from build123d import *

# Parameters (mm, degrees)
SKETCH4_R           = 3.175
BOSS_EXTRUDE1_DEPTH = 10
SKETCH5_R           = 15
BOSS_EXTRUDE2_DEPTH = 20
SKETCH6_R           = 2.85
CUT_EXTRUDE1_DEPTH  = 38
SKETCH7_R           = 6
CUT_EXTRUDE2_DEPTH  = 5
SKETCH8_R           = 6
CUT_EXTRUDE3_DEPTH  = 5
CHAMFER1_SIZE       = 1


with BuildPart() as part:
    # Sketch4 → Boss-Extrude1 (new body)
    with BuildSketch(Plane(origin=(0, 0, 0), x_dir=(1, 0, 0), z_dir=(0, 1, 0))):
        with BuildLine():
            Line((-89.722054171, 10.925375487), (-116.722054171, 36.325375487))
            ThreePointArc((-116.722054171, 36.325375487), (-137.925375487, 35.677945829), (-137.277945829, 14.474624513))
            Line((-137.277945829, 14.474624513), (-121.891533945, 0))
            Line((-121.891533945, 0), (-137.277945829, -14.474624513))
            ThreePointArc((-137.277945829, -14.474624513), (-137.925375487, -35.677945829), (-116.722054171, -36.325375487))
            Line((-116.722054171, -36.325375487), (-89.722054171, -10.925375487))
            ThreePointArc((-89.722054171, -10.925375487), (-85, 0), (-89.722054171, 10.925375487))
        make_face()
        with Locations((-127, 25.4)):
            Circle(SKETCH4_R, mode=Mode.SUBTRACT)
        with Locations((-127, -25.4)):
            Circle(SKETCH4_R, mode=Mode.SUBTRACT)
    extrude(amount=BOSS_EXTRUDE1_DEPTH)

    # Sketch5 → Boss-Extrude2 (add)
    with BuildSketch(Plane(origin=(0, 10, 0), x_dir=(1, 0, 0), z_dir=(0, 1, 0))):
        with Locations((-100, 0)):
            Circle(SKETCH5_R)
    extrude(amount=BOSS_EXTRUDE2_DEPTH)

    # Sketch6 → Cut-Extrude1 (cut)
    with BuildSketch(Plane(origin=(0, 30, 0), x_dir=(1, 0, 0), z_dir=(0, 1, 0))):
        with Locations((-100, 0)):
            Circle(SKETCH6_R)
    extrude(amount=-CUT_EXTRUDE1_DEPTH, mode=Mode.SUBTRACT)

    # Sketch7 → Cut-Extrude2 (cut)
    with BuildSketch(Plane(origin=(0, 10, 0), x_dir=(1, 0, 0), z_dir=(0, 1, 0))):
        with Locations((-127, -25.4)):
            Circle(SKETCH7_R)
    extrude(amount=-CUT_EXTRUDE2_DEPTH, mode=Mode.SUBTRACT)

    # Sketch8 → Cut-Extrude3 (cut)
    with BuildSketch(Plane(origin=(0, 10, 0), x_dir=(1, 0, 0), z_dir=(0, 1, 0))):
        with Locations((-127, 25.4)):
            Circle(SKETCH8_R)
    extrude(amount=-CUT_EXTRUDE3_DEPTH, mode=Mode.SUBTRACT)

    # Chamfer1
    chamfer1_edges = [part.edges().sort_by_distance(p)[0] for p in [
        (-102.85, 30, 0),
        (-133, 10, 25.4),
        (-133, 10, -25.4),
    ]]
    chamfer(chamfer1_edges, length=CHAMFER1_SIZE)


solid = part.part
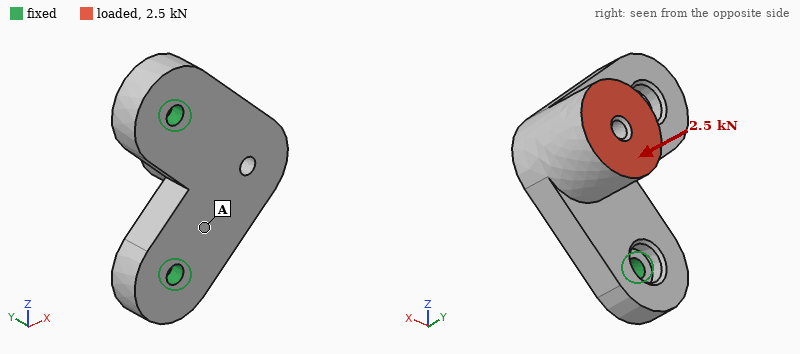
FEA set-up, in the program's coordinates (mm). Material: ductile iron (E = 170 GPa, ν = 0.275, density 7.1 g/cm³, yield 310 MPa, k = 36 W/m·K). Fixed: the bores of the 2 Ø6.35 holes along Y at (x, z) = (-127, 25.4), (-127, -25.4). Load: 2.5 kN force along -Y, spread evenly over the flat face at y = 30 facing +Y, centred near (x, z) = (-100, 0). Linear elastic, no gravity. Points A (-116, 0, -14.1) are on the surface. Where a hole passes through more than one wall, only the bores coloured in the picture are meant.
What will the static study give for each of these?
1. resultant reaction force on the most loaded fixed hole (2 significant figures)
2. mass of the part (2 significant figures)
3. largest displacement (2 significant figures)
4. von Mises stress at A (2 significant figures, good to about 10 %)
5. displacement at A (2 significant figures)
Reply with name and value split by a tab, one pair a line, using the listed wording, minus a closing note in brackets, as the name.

resultant reaction force on the most loaded fixed hole	1.3 kN
mass of the part	290 g
largest displacement	0.12 mm
von Mises stress at A	44 MPa
displacement at A	0.023 mm
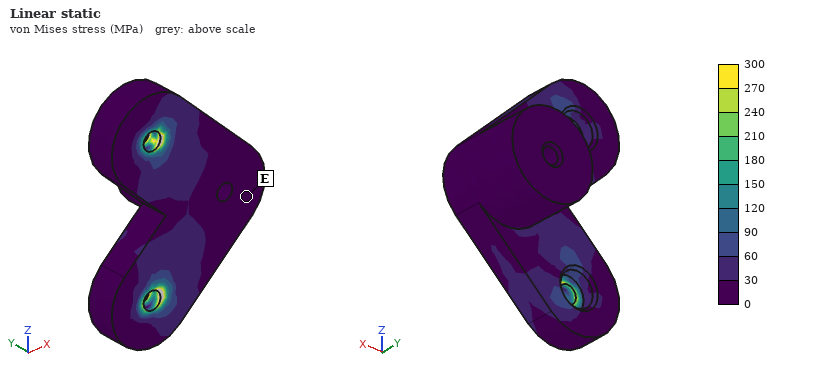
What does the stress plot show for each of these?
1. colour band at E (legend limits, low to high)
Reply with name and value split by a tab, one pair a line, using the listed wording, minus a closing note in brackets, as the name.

colour band at E	0 to 30 MPa
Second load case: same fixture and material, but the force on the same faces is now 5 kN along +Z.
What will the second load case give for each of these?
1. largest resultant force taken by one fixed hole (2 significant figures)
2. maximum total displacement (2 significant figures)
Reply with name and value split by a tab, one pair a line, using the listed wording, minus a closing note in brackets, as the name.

largest resultant force taken by one fixed hole	4.5 kN
maximum total displacement	46 µm
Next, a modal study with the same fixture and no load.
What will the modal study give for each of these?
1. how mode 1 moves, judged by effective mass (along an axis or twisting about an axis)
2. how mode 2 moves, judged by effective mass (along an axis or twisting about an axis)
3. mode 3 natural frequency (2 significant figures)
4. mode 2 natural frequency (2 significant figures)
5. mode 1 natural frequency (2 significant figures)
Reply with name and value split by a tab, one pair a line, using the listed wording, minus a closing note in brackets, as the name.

how mode 1 moves, judged by effective mass	along Y
how mode 2 moves, judged by effective mass	along Z
mode 3 natural frequency	8900 Hz
mode 2 natural frequency	7200 Hz
mode 1 natural frequency	2100 Hz
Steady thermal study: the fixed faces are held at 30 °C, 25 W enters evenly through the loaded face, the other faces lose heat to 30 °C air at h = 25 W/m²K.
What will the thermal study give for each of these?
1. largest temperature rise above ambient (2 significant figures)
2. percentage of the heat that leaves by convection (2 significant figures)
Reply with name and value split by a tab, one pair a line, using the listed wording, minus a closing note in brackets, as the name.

largest temperature rise above ambient	58 K
percentage of the heat that leaves by convection	23 %
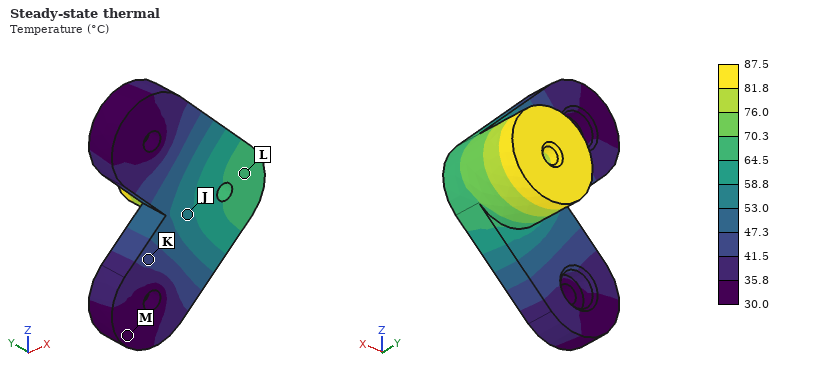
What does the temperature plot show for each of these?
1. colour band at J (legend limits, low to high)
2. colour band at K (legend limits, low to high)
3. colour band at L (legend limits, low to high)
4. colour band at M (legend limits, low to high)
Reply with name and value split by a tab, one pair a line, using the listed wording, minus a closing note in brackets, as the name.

colour band at J	53.0 to 58.8 °C
colour band at K	41.5 to 47.3 °C
colour band at L	64.5 to 70.3 °C
colour band at M	30.0 to 35.8 °C
